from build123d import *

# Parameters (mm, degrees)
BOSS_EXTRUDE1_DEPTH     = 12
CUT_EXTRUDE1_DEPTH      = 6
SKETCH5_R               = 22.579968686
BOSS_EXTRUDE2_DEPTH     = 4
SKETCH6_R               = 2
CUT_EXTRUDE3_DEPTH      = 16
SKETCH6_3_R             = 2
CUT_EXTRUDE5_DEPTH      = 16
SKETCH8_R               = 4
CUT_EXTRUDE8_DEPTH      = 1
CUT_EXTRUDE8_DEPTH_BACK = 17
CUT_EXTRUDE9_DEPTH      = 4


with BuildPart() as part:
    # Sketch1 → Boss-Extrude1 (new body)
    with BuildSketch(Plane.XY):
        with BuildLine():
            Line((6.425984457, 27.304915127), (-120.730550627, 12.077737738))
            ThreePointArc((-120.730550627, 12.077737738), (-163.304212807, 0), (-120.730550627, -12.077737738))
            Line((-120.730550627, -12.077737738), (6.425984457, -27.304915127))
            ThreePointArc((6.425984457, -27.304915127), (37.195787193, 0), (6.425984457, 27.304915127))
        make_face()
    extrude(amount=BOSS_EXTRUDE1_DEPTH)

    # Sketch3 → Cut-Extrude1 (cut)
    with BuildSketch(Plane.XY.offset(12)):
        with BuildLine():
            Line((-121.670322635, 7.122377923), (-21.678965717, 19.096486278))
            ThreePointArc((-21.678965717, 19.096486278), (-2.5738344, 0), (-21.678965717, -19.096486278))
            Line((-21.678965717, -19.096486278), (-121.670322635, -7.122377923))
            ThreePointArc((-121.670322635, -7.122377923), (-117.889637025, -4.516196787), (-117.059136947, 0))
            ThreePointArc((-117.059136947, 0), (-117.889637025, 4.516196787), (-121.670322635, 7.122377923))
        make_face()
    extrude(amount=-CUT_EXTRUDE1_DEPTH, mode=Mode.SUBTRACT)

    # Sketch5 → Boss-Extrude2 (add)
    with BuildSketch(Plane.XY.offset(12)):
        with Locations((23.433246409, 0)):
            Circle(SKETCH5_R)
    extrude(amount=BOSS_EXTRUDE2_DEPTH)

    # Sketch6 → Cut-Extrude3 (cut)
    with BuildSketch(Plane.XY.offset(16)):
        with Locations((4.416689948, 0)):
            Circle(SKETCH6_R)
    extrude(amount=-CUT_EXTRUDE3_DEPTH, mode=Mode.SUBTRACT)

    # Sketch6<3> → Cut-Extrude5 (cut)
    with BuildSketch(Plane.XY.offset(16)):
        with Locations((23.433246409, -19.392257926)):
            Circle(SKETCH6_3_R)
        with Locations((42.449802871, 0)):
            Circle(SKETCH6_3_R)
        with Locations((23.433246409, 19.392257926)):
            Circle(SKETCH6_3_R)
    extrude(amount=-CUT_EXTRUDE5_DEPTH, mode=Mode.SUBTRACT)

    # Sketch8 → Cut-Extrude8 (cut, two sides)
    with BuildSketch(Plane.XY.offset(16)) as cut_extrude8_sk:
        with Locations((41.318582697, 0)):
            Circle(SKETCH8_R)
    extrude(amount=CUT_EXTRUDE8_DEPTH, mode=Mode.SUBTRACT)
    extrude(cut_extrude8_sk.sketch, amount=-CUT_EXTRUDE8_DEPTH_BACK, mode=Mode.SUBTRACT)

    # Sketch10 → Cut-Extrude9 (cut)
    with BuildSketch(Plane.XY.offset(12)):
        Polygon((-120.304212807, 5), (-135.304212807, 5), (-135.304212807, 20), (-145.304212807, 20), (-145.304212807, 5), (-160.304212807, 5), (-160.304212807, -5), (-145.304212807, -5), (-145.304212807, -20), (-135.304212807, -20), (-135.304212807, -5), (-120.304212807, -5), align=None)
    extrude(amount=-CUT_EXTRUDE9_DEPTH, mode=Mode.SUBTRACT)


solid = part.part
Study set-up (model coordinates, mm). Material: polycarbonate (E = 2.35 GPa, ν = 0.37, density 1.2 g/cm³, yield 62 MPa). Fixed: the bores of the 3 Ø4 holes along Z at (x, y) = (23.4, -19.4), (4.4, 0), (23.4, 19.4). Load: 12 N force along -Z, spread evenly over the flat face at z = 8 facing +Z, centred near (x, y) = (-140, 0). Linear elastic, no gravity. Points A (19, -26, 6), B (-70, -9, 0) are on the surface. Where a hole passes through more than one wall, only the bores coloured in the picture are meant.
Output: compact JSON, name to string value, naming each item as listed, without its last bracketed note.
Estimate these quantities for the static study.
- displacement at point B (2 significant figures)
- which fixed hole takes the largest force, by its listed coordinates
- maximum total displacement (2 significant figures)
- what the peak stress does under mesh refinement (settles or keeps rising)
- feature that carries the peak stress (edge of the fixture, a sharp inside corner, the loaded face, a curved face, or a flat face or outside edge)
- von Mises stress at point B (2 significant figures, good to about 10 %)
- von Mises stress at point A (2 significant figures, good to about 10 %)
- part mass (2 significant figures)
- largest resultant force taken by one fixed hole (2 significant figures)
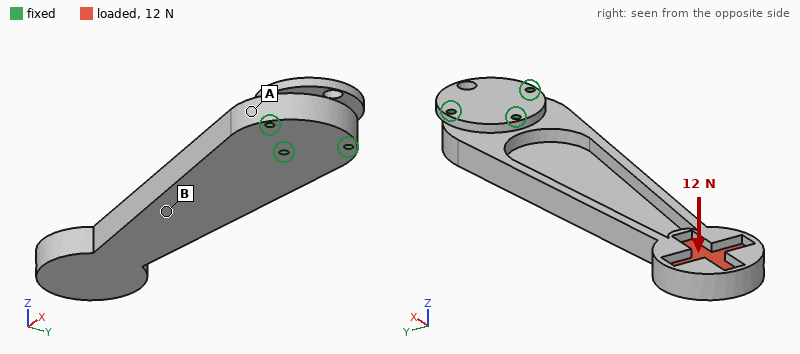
{"displacement at point B": "0.54 mm", "which fixed hole takes the largest force, by its listed coordinates": "(4.4, 0)", "maximum total displacement": "2.2 mm", "what the peak stress does under mesh refinement": "keeps rising", "feature that carries the peak stress": "edge of the fixture", "von Mises stress at point B": "1.5 MPa", "von Mises stress at point A": "0.46 MPa", "part mass": "96 g", "largest resultant force taken by one fixed hole": "68 N"}
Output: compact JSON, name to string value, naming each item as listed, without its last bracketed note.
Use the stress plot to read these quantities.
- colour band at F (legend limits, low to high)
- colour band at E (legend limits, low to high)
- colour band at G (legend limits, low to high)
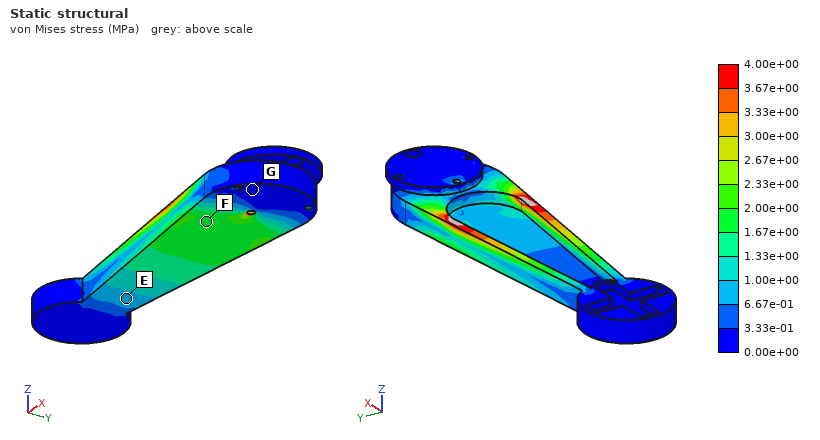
{"colour band at F": "1.67e+00 to 2.00e+00 MPa", "colour band at E": "6.67e-01 to 1.00e+00 MPa", "colour band at G": "0.00e+00 to 3.33e-01 MPa"}
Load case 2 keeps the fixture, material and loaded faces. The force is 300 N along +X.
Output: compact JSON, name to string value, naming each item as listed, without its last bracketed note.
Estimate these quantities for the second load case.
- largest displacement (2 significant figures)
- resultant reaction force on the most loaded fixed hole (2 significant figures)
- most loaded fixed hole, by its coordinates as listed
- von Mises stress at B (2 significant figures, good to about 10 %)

{"largest displacement": "2.4 mm", "resultant reaction force on the most loaded fixed hole": "110 N", "most loaded fixed hole, by its coordinates as listed": "(4.4, 0)", "von Mises stress at B": "0.86 MPa"}
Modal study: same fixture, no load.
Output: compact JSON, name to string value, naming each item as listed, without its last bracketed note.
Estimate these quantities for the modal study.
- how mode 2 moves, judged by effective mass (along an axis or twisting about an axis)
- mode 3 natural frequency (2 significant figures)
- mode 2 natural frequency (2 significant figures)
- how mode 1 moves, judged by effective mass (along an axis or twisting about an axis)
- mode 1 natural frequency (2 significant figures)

{"how mode 2 moves, judged by effective mass": "along Y", "mode 3 natural frequency": "420 Hz", "mode 2 natural frequency": "330 Hz", "how mode 1 moves, judged by effective mass": "along Z", "mode 1 natural frequency": "83 Hz"}
